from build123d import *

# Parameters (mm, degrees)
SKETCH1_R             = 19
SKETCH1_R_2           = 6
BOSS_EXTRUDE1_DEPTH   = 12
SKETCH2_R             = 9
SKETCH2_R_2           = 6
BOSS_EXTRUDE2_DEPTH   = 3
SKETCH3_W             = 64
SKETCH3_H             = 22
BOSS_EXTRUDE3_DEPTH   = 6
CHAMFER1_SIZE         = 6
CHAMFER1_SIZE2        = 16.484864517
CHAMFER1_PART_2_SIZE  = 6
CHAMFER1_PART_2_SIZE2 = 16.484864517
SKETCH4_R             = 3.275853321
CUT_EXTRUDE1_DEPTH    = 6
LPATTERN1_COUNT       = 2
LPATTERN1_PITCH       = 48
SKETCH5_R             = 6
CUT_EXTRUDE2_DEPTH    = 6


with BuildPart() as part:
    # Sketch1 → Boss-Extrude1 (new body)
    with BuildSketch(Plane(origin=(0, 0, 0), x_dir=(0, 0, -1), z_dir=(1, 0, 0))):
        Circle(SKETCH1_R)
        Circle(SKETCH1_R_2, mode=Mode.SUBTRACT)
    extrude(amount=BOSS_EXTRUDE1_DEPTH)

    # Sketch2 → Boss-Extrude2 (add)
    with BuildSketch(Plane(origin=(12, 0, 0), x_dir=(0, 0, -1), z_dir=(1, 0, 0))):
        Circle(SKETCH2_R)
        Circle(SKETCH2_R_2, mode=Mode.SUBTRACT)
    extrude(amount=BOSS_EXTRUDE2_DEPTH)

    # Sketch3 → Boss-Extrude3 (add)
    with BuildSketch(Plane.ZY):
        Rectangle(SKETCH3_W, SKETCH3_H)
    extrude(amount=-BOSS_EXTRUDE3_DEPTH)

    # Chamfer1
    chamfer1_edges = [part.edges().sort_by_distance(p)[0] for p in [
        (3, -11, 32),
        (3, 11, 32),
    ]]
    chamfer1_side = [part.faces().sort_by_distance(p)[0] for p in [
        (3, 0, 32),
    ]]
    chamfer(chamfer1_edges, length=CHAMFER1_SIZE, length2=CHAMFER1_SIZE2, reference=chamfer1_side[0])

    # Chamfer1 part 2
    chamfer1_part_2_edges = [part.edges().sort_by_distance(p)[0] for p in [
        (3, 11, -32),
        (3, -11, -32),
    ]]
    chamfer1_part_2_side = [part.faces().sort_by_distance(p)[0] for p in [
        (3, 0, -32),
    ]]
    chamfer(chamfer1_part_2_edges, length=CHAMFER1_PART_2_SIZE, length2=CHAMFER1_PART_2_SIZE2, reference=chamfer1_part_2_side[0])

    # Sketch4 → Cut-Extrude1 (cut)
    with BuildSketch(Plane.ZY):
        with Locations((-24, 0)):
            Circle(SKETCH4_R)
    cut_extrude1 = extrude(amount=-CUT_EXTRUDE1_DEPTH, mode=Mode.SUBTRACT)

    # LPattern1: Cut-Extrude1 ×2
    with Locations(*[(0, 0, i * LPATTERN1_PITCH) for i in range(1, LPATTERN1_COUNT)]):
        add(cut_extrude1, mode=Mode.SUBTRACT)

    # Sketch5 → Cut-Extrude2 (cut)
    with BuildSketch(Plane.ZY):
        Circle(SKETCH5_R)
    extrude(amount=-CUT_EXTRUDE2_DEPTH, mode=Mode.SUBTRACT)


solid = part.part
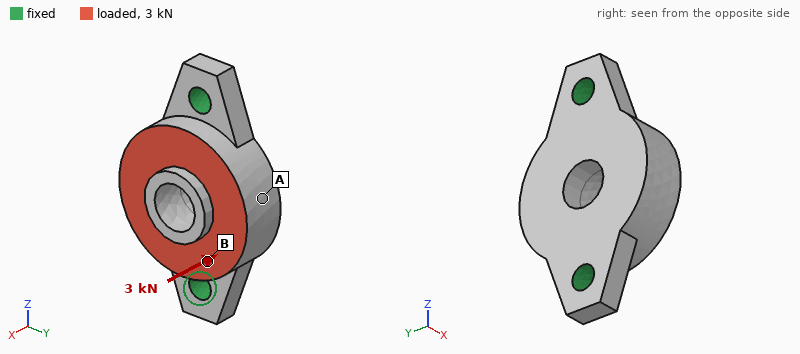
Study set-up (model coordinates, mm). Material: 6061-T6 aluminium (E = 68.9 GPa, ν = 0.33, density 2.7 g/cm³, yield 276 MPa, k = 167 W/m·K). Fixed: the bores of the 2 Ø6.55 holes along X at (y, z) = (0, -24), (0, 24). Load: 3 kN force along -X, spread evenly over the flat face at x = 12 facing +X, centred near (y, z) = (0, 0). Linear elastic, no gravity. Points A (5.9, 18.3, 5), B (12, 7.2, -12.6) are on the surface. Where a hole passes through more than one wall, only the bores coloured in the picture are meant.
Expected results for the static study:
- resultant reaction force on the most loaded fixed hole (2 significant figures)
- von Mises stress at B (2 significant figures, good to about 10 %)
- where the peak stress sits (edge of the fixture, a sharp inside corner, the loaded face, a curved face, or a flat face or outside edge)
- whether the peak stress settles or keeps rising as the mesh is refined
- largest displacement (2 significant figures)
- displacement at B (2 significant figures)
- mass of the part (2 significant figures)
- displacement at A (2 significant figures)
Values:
1.8 kN
18 MPa
edge of the fixture
keeps rising
19 µm
11 µm
40 g
18 µm
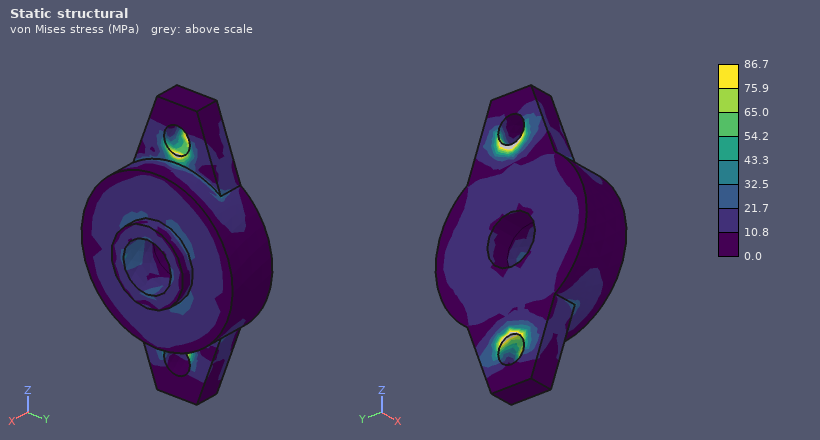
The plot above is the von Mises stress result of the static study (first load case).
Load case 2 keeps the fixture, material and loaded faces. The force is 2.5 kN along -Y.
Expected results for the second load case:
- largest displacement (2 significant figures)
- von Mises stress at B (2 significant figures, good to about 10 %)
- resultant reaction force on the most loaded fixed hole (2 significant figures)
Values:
48 µm
14 MPa
1.3 kN
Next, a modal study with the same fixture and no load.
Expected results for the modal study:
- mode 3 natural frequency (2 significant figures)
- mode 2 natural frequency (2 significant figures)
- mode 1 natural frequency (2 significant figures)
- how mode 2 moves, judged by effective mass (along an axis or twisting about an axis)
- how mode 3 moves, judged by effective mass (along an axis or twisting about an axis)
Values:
21 kHz
13 kHz
8000 Hz
along X
along Y
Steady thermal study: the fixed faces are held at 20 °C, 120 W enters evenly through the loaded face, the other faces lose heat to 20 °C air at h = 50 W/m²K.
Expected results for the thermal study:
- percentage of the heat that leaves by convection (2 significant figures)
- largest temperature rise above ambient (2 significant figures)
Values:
4.0 %
36 K
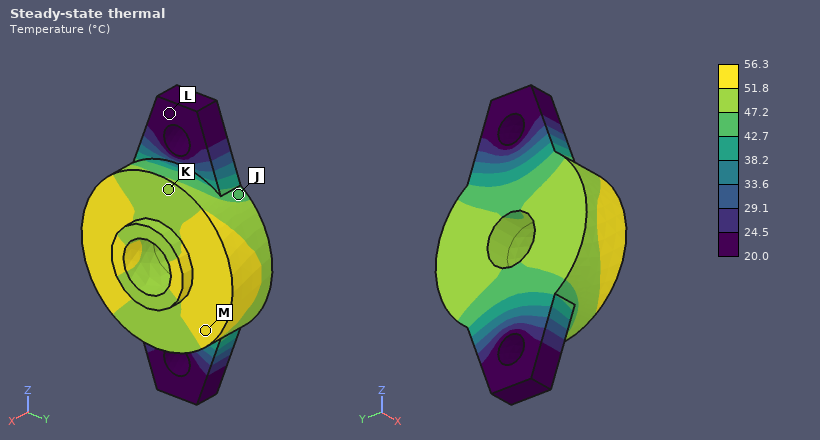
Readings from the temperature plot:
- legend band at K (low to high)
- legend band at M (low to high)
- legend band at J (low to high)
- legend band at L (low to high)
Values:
47.2 to 51.8 °C
51.8 to 56.3 °C
42.7 to 47.2 °C
20.0 to 24.5 °C
